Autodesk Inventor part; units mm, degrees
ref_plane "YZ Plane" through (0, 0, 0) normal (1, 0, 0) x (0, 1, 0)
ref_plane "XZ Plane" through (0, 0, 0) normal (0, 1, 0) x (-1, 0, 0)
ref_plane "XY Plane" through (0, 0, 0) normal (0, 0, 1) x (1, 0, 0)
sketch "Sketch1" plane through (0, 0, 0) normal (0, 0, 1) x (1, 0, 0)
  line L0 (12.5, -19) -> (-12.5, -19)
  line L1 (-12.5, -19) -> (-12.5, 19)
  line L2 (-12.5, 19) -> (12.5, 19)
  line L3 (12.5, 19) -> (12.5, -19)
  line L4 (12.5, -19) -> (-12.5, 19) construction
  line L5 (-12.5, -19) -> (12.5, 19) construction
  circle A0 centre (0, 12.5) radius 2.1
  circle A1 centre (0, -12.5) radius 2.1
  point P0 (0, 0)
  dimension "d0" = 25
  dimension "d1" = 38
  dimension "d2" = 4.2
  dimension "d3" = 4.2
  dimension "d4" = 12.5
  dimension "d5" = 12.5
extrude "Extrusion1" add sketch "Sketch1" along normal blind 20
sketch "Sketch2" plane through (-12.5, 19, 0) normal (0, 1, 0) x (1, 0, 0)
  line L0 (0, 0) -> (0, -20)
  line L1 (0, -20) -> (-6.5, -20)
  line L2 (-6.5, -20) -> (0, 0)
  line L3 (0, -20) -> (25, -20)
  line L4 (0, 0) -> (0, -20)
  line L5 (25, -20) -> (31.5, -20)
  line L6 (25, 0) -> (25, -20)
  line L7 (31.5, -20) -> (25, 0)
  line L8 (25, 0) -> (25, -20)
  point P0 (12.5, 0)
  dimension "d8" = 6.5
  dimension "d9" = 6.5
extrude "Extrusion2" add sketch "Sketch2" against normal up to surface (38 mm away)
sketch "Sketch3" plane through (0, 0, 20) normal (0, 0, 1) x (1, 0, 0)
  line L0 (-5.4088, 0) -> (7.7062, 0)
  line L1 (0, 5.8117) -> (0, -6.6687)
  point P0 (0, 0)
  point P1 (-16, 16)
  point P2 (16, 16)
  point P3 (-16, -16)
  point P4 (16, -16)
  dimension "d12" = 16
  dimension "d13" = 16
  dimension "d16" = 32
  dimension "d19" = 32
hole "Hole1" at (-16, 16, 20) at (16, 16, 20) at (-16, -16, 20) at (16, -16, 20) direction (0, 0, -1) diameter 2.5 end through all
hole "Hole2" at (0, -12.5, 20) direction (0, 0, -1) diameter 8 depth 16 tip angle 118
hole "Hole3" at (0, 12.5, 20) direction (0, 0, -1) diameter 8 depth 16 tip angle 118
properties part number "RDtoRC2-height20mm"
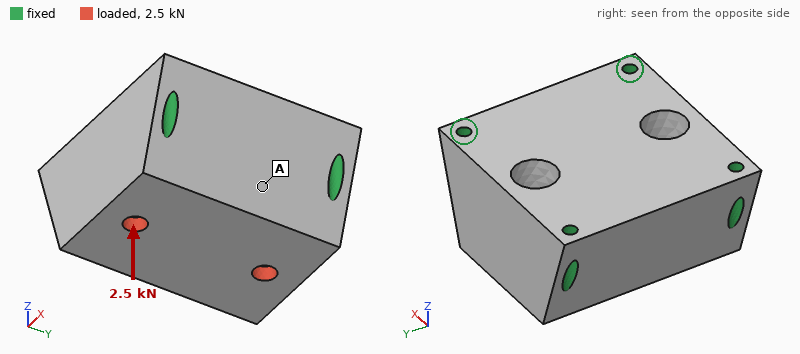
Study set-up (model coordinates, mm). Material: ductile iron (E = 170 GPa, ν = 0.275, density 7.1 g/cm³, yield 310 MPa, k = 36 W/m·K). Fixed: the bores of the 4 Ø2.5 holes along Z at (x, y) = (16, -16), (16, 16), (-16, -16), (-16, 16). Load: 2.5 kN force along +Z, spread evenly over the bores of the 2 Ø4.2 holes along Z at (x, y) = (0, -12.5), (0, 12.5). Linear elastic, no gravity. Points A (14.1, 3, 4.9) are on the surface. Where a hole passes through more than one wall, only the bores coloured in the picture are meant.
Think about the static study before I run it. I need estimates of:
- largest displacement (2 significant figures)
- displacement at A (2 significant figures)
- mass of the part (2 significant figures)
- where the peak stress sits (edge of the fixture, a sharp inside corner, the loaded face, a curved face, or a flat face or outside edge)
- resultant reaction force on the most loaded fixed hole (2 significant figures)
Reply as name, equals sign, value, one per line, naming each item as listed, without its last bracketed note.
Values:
largest displacement = 3.2 µm
displacement at A = 0.62 µm
mass of the part = 160 g
where the peak stress sits = the loaded face
resultant reaction force on the most loaded fixed hole = 690 N
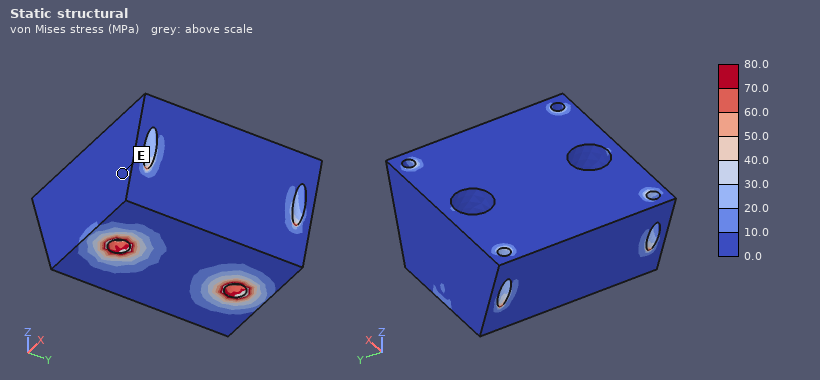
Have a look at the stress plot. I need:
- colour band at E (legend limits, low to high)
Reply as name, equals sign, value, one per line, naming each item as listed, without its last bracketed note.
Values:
colour band at E = 0.0 to 10.0 MPa
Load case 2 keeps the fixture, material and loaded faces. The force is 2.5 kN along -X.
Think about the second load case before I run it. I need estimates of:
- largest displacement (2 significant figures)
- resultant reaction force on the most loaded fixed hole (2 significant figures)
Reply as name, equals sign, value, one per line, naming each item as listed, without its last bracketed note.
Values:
largest displacement = 1.8 µm
resultant reaction force on the most loaded fixed hole = 790 N
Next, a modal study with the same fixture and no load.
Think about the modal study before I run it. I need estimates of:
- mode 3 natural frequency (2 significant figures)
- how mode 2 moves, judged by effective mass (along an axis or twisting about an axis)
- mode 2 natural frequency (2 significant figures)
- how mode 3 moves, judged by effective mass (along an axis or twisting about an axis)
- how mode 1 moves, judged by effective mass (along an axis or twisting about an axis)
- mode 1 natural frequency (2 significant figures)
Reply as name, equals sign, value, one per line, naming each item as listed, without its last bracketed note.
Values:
mode 3 natural frequency = 29 kHz
how mode 2 moves, judged by effective mass = along Y
mode 2 natural frequency = 28 kHz
how mode 3 moves, judged by effective mass = along X
how mode 1 moves, judged by effective mass = along Z
mode 1 natural frequency = 23 kHz
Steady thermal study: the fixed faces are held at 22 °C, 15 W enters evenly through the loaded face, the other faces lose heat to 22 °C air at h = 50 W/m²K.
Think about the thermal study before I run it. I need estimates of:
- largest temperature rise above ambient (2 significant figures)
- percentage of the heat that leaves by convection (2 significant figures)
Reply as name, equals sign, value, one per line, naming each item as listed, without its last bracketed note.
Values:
largest temperature rise above ambient = 22 K
percentage of the heat that leaves by convection = 11 %
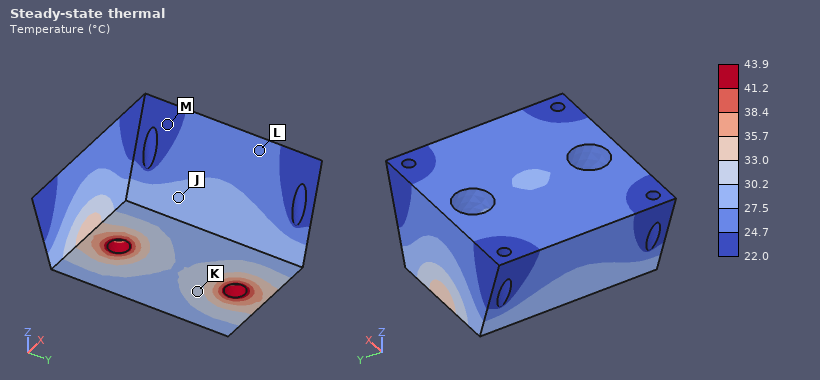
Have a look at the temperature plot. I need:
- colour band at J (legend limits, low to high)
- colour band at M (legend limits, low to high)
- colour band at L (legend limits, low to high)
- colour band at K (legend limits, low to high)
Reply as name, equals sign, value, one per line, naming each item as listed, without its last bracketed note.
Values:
colour band at J = 27.5 to 30.2 °C
colour band at M = 22.0 to 24.7 °C
colour band at L = 24.7 to 27.5 °C
colour band at K = 30.2 to 33.0 °C
